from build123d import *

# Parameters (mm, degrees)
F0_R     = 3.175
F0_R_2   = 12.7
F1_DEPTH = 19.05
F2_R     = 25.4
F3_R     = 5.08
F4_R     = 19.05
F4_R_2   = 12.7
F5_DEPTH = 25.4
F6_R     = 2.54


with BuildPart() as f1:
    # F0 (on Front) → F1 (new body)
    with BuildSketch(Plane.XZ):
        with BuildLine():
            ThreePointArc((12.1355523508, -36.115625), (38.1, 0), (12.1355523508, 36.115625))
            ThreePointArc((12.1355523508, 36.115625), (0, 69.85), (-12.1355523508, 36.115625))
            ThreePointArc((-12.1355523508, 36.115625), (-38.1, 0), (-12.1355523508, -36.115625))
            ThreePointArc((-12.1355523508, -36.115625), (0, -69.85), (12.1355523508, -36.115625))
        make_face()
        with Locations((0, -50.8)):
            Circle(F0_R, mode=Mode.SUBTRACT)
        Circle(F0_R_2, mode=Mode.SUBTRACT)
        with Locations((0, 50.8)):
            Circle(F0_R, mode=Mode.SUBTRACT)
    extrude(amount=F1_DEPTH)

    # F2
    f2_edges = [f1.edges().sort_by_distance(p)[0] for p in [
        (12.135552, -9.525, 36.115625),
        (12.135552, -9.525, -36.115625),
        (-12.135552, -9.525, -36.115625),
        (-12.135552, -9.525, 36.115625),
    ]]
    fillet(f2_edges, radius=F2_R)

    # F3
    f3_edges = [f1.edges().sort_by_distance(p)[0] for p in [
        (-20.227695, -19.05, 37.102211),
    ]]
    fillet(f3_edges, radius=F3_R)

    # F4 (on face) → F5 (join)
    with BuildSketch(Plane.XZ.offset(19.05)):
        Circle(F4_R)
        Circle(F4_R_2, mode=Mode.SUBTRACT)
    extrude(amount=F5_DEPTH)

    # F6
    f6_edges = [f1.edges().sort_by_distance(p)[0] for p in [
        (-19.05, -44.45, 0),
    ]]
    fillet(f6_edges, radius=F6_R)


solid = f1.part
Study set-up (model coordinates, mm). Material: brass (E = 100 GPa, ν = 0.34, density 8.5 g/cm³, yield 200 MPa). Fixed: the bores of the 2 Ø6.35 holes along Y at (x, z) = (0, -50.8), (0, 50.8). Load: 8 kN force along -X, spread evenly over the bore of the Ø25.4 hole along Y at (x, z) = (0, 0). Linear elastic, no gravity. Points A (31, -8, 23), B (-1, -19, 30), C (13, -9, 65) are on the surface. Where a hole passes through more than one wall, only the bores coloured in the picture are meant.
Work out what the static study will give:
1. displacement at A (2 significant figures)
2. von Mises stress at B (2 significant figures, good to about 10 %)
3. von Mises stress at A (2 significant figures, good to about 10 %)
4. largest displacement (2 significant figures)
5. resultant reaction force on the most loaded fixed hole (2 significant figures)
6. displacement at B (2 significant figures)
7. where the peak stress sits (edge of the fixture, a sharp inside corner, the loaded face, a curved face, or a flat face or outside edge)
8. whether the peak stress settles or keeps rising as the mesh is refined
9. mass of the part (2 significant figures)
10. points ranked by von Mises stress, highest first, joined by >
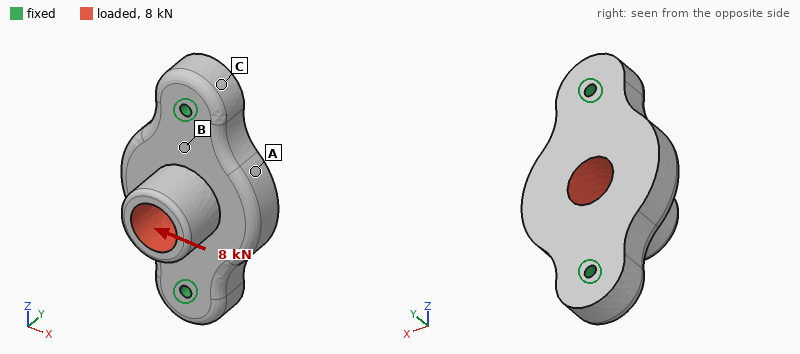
21 µm
23 MPa
12 MPa
44 µm
4.0 kN
11 µm
edge of the fixture
keeps rising
1.1 kg
B > A > C
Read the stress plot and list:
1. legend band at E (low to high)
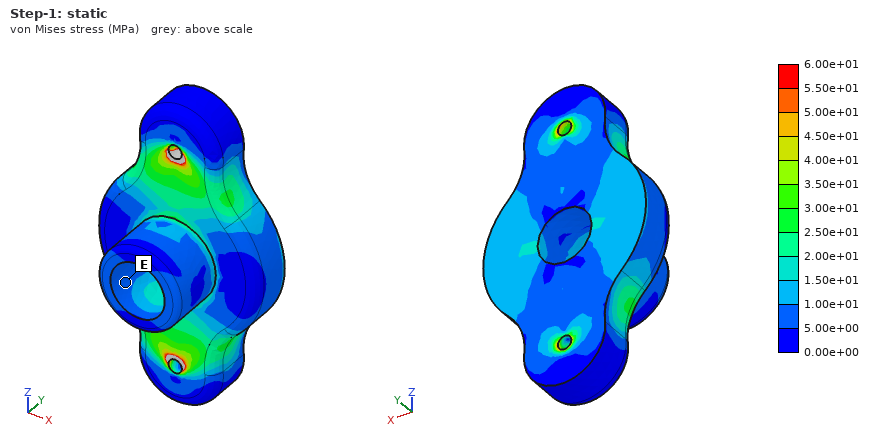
5.00e+00 to 1.00e+01 MPa
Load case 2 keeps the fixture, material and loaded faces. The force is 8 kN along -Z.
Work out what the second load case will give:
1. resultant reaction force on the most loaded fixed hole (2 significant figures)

4.2 kN
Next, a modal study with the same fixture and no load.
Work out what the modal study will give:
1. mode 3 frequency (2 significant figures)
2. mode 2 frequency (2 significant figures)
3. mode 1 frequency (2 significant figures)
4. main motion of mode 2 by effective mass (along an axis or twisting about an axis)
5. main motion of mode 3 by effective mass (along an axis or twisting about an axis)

6000 Hz
3700 Hz
3100 Hz
along Y
along X
